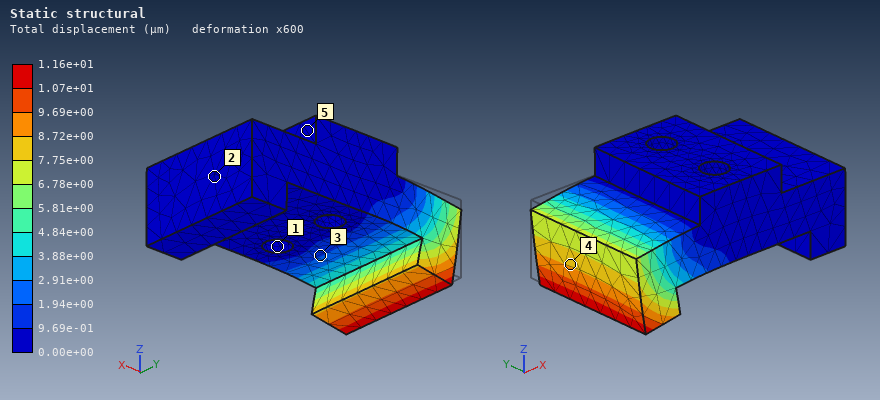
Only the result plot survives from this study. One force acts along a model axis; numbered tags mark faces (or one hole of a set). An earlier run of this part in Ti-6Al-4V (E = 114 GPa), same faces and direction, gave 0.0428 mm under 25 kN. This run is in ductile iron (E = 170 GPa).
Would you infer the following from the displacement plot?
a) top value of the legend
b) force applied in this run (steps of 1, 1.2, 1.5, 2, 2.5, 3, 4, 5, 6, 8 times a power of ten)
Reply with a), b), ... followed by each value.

a) 1.16e+01 µm
b) 10 kN
